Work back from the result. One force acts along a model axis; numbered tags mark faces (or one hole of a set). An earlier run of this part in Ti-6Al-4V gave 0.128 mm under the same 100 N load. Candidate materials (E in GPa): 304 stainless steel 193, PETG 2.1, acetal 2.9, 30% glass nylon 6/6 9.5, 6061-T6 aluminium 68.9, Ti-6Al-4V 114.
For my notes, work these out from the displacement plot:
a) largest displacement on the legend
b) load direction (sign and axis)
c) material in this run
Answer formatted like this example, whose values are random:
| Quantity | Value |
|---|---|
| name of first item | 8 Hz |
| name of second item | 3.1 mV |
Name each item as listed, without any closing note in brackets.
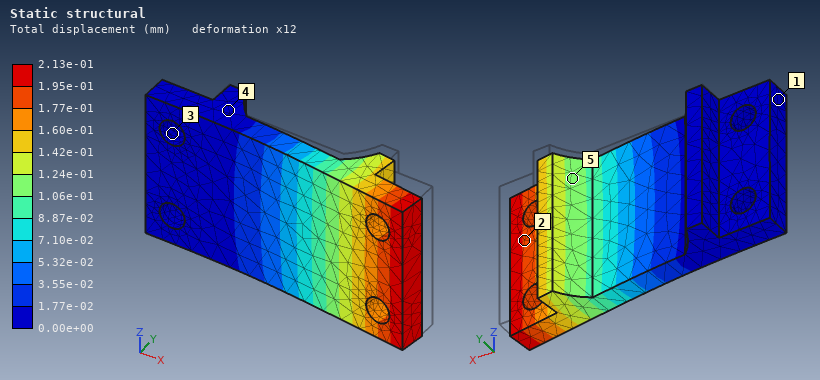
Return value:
| Quantity | Value |
|---|---|
| largest displacement on the legend | 2.13e-01 mm |
| load direction | -Y |
| material in this run | 6061-T6 aluminium |
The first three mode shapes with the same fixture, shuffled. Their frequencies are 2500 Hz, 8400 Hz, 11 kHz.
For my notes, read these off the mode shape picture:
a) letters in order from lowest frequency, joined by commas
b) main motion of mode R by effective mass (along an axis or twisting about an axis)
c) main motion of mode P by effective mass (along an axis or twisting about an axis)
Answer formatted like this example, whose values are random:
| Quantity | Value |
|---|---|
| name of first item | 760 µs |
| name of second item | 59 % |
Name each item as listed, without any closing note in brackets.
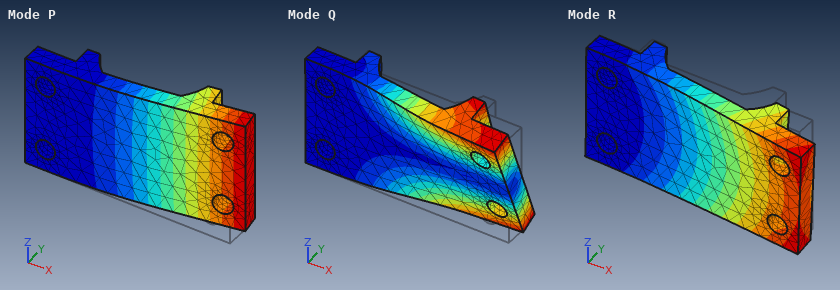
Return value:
| Quantity | Value |
|---|---|
| letters in order from lowest frequency, joined by commas | P, Q, R |
| main motion of mode R by effective mass | along Z |
| main motion of mode P by effective mass | along Y |
